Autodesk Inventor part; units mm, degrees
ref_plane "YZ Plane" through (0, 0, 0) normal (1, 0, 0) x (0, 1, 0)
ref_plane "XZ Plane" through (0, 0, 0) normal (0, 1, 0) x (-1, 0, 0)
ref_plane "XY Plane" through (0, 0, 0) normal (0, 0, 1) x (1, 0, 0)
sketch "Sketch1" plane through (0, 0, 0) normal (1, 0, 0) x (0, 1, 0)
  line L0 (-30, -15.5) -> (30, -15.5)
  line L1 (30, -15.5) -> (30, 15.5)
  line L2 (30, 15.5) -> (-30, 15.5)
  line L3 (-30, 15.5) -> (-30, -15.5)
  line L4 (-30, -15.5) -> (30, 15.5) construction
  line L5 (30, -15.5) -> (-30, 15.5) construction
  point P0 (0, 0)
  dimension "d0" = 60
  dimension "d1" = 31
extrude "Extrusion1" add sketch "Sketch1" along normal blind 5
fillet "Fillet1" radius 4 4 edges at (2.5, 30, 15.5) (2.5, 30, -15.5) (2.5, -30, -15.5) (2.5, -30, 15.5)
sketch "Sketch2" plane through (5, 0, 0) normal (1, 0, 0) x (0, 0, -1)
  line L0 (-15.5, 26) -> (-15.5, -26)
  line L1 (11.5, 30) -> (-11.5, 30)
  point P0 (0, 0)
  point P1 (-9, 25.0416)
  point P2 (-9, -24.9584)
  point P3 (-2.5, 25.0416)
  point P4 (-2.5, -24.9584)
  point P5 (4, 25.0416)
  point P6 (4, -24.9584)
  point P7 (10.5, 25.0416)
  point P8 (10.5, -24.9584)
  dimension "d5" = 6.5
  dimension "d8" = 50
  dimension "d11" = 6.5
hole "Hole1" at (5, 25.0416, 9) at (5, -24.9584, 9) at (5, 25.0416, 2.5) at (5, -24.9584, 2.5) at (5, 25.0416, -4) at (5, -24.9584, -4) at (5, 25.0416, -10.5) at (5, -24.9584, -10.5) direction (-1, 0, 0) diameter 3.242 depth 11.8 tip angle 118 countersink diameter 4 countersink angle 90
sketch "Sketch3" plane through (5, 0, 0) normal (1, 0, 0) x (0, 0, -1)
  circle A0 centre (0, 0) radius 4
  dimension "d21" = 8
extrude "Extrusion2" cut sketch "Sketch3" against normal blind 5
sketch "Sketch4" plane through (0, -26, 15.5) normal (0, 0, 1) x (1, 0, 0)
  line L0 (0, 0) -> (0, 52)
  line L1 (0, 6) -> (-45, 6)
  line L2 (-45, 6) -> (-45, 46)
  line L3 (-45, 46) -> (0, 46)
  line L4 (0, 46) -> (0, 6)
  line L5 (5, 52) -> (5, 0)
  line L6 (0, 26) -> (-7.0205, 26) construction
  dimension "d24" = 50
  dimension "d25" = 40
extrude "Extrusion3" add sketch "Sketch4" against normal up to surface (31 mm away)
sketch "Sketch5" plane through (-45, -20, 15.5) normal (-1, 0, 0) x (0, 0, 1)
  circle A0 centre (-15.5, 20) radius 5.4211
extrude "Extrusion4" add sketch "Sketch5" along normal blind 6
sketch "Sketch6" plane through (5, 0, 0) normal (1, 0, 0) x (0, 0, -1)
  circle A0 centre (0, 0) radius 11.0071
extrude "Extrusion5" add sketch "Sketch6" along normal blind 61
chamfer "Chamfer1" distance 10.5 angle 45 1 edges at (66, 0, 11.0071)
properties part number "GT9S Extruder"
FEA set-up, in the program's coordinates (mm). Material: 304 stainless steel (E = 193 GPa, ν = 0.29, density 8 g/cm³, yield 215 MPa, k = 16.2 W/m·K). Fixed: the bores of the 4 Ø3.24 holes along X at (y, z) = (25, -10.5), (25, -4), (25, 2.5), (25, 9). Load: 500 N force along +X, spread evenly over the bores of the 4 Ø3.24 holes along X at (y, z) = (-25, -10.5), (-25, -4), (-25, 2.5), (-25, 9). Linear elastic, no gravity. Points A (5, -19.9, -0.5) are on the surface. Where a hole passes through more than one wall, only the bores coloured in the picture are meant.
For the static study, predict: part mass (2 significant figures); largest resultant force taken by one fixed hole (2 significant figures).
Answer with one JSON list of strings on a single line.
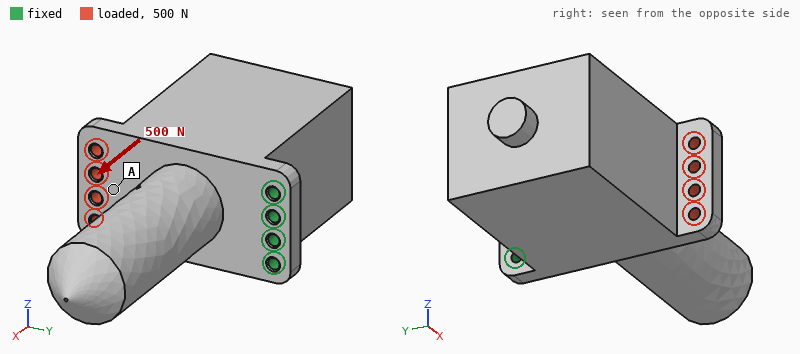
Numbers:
["680 g", "200 N"]
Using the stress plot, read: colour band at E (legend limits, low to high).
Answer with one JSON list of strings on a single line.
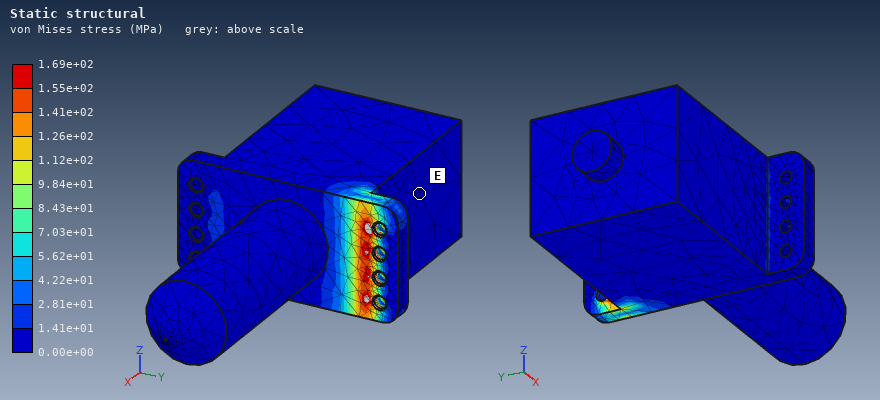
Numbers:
["0.00e+00 to 1.41e+01 MPa"]
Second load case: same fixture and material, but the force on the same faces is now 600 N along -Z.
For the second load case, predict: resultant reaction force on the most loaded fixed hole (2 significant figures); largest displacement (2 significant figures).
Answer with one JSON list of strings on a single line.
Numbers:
["1.3 kN", "12 µm"]
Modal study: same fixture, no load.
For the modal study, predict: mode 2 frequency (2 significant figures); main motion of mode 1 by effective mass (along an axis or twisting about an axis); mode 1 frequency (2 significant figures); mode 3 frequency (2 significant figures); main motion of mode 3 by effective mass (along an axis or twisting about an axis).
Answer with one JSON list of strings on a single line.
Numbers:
["1500 Hz", "along X", "490 Hz", "2700 Hz", "along Z"]
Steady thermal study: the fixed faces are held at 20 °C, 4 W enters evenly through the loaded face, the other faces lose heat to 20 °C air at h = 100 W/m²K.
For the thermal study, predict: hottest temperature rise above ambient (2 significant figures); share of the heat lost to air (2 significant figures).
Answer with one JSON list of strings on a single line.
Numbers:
["19 K", "90 %"]
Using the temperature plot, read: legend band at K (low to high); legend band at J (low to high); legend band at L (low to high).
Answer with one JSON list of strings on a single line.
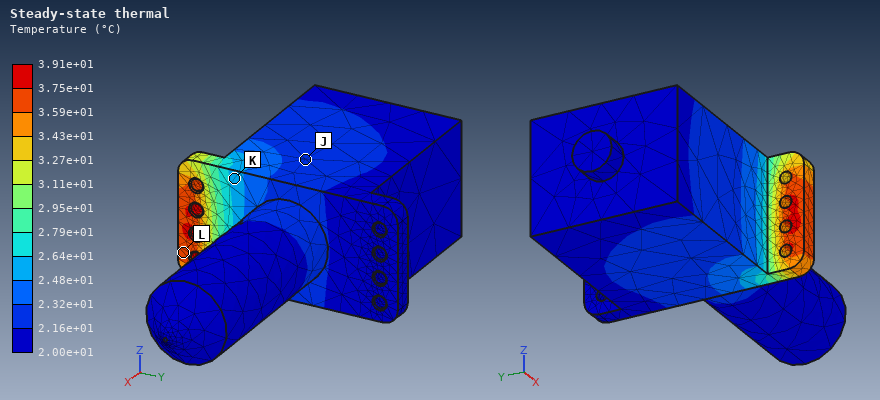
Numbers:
["2.48e+01 to 2.64e+01 °C", "2.16e+01 to 2.32e+01 °C", "3.59e+01 to 3.75e+01 °C"]
